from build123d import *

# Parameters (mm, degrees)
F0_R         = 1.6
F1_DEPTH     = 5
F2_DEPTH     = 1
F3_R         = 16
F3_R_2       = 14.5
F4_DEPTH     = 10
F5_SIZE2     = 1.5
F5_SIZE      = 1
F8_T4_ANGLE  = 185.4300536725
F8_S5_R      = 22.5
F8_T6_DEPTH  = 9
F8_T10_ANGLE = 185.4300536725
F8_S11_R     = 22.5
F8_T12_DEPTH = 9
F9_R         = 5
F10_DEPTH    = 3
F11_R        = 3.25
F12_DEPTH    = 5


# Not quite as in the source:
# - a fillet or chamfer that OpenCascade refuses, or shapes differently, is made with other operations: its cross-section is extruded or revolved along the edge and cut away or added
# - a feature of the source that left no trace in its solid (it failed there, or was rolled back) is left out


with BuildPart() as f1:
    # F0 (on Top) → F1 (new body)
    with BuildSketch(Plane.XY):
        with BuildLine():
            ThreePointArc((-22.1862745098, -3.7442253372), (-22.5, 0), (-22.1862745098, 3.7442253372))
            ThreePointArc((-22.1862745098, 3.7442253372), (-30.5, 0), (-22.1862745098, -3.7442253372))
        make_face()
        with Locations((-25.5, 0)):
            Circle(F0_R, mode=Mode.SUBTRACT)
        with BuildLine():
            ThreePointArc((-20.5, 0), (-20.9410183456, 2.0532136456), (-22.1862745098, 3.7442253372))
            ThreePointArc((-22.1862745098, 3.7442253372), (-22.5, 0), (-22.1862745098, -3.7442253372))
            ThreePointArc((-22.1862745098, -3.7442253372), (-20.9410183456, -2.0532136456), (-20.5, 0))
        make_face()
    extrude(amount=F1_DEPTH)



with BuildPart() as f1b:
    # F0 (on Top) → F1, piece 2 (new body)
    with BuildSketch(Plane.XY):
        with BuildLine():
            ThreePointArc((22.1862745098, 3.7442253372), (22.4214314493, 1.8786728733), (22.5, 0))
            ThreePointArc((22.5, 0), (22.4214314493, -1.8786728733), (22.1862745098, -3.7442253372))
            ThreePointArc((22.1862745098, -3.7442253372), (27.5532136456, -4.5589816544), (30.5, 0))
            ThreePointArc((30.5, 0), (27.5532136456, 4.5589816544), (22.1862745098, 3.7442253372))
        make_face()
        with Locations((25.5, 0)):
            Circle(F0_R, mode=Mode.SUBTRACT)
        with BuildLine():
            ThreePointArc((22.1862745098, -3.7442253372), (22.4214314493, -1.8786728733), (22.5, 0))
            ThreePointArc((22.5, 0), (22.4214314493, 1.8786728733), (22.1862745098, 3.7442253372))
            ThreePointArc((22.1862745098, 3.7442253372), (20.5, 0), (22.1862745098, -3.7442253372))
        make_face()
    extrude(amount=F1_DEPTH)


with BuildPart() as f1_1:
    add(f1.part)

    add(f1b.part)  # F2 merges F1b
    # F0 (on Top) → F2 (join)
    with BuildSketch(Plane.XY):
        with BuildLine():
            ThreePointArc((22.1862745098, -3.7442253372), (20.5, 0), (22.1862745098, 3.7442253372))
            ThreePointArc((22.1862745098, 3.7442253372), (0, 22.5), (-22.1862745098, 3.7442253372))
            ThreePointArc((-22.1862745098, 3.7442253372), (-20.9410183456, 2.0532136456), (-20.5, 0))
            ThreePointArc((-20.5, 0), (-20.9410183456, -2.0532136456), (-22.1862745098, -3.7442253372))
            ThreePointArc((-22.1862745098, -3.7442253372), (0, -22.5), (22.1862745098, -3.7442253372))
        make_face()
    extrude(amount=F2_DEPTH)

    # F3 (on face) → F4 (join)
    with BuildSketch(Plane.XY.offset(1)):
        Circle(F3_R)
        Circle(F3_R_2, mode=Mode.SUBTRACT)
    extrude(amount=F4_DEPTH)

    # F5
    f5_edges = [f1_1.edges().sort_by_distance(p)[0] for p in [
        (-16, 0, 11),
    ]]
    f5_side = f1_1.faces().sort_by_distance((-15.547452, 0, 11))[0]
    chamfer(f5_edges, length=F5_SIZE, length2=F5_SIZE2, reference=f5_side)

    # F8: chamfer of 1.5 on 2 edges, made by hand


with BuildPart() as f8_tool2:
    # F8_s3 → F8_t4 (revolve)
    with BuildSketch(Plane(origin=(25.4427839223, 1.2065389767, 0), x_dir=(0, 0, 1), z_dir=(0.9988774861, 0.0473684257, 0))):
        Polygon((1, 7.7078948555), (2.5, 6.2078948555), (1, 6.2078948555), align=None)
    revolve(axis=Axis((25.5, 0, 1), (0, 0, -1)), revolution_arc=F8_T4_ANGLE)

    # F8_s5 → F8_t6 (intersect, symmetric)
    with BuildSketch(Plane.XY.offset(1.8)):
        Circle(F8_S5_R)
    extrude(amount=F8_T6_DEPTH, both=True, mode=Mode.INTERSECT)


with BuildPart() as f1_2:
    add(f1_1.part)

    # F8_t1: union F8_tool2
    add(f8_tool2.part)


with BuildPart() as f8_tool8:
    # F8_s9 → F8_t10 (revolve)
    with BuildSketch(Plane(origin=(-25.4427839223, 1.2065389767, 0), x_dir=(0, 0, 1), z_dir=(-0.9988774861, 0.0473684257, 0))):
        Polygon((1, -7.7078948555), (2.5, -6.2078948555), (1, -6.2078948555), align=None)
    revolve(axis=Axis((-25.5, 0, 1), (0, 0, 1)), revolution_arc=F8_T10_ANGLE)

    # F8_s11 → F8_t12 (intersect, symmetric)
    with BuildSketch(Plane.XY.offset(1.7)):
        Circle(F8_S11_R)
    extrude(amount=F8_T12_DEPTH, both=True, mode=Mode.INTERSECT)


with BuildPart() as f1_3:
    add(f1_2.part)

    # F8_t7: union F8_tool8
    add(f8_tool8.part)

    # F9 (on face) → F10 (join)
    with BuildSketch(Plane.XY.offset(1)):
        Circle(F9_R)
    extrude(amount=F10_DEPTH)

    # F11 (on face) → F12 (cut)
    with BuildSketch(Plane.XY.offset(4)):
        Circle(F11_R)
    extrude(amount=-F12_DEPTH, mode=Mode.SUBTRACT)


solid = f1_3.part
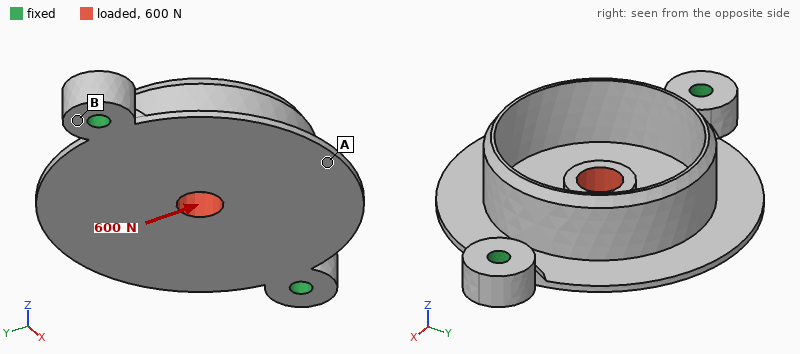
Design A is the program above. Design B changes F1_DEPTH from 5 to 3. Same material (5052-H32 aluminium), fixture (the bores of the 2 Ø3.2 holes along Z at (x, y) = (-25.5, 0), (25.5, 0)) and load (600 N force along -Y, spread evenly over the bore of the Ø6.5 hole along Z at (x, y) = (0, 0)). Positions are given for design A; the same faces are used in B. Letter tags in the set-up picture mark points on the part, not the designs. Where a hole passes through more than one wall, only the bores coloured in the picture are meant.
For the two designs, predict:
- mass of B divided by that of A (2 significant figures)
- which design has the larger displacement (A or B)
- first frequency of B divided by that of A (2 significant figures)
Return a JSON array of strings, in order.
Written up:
["0.93", "B", "0.94"]
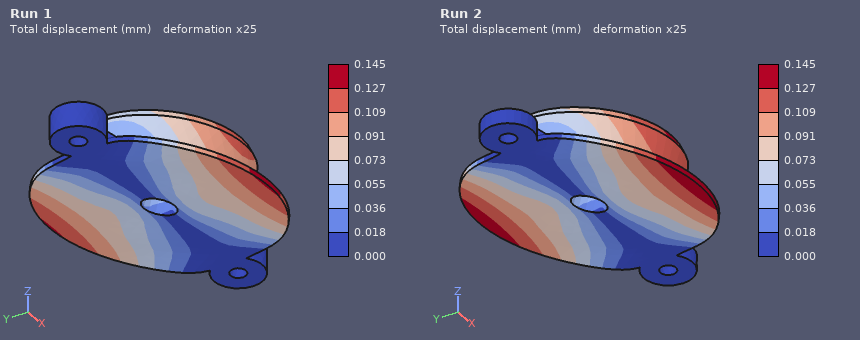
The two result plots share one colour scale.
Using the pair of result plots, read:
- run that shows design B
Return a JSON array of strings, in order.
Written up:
["Run 2"]
